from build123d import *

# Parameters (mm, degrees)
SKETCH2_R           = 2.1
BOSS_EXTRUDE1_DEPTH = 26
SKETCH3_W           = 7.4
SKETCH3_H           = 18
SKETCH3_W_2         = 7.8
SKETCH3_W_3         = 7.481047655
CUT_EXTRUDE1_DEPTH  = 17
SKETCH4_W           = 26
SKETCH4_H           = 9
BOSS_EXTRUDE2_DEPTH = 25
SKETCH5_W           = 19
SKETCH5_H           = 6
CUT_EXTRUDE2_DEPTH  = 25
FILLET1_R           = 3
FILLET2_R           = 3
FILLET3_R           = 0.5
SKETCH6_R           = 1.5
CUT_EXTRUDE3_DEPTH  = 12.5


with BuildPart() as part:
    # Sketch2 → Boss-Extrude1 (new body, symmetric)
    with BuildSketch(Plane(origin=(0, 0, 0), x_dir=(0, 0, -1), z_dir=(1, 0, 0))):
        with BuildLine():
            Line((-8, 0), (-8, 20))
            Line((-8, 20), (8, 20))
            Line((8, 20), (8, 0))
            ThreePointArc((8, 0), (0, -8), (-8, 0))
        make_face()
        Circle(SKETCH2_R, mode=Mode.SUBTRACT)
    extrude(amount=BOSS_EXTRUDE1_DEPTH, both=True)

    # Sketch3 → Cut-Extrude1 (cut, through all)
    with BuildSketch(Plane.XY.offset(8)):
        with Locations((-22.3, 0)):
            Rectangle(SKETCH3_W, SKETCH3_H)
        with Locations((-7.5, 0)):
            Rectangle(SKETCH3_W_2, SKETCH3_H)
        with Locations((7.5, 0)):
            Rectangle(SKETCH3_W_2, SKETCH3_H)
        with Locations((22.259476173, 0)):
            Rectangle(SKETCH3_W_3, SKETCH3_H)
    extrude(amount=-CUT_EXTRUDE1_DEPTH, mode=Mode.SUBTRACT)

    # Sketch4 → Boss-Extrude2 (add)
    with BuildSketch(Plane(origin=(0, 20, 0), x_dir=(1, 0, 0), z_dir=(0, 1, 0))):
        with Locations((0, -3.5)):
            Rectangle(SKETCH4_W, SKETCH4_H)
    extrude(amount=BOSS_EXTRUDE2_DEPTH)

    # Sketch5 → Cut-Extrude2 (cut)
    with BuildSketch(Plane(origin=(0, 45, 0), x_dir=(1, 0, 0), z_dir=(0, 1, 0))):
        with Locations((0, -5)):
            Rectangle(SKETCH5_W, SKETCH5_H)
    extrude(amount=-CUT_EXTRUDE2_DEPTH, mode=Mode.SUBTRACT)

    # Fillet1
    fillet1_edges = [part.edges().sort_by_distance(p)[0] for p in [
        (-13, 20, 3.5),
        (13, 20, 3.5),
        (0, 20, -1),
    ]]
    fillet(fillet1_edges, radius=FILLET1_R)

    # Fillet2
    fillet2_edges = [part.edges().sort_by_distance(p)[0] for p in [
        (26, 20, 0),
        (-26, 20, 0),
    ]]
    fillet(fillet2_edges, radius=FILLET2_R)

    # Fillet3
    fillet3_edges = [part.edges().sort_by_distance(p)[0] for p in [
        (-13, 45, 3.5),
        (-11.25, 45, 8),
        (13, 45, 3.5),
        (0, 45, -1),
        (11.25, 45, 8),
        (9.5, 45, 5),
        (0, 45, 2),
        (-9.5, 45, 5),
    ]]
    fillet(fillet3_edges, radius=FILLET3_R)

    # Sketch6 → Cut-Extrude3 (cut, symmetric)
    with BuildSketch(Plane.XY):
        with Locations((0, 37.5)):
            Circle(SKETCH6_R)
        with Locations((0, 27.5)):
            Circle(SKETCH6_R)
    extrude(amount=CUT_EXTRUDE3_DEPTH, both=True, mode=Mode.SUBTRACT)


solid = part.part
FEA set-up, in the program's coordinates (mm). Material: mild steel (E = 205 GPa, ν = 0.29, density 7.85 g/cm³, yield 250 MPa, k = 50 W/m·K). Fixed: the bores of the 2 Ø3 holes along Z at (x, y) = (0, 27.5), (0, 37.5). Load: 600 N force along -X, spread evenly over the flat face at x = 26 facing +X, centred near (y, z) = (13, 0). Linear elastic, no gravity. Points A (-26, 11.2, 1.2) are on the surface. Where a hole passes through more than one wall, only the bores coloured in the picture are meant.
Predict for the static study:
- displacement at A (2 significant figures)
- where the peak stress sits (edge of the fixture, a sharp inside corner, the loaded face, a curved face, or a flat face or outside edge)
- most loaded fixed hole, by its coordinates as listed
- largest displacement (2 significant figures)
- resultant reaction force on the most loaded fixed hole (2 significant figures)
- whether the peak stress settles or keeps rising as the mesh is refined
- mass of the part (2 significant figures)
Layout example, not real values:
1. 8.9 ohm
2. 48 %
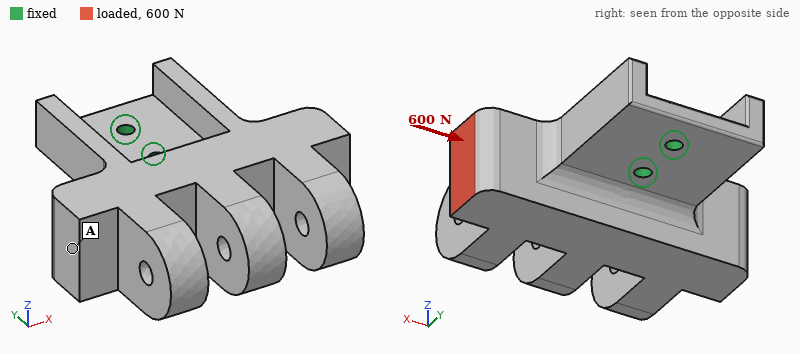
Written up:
1. 8.5 µm
2. edge of the fixture
3. (0, 27.5)
4. 12 µm
5. 1.2 kN
6. keeps rising
7. 130 g
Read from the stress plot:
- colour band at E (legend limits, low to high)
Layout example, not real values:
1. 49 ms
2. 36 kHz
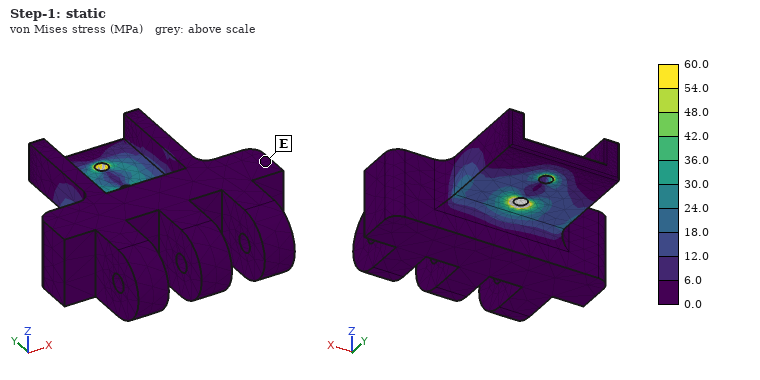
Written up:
1. 0.0 to 6.0 MPa
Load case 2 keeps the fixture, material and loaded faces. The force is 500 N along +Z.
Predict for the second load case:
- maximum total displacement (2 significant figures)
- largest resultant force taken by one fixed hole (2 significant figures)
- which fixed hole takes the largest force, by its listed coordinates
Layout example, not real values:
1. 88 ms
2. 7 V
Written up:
1. 0.11 mm
2. 880 N
3. (0, 27.5)
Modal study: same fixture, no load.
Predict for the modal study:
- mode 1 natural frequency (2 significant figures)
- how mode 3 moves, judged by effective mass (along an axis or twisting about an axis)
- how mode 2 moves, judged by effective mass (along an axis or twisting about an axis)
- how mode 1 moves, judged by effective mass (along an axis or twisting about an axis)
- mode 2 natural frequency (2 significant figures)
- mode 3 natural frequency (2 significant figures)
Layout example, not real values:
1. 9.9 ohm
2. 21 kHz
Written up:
1. 1900 Hz
2. along X
3. twisting about Y
4. along Z
5. 2000 Hz
6. 3600 Hz
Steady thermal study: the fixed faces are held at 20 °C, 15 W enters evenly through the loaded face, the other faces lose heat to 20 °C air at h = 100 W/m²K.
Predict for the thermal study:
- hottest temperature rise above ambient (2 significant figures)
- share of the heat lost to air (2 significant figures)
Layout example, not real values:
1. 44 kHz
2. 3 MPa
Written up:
1. 46 K
2. 63 %
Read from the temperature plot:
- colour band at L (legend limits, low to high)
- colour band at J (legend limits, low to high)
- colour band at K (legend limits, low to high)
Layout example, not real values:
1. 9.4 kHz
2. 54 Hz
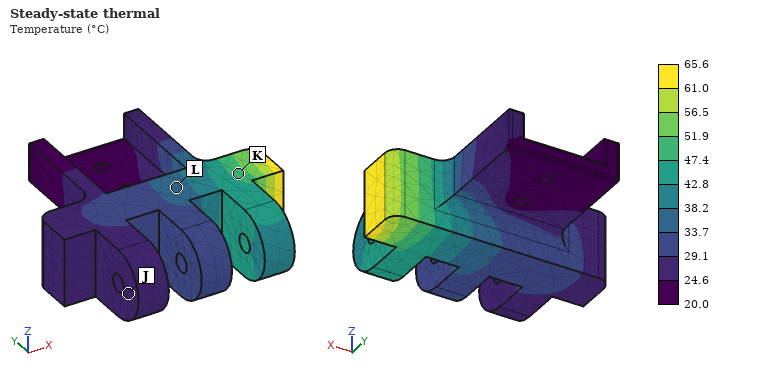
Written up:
1. 33.7 to 38.2 °C
2. 24.6 to 29.1 °C
3. 47.4 to 51.9 °C
